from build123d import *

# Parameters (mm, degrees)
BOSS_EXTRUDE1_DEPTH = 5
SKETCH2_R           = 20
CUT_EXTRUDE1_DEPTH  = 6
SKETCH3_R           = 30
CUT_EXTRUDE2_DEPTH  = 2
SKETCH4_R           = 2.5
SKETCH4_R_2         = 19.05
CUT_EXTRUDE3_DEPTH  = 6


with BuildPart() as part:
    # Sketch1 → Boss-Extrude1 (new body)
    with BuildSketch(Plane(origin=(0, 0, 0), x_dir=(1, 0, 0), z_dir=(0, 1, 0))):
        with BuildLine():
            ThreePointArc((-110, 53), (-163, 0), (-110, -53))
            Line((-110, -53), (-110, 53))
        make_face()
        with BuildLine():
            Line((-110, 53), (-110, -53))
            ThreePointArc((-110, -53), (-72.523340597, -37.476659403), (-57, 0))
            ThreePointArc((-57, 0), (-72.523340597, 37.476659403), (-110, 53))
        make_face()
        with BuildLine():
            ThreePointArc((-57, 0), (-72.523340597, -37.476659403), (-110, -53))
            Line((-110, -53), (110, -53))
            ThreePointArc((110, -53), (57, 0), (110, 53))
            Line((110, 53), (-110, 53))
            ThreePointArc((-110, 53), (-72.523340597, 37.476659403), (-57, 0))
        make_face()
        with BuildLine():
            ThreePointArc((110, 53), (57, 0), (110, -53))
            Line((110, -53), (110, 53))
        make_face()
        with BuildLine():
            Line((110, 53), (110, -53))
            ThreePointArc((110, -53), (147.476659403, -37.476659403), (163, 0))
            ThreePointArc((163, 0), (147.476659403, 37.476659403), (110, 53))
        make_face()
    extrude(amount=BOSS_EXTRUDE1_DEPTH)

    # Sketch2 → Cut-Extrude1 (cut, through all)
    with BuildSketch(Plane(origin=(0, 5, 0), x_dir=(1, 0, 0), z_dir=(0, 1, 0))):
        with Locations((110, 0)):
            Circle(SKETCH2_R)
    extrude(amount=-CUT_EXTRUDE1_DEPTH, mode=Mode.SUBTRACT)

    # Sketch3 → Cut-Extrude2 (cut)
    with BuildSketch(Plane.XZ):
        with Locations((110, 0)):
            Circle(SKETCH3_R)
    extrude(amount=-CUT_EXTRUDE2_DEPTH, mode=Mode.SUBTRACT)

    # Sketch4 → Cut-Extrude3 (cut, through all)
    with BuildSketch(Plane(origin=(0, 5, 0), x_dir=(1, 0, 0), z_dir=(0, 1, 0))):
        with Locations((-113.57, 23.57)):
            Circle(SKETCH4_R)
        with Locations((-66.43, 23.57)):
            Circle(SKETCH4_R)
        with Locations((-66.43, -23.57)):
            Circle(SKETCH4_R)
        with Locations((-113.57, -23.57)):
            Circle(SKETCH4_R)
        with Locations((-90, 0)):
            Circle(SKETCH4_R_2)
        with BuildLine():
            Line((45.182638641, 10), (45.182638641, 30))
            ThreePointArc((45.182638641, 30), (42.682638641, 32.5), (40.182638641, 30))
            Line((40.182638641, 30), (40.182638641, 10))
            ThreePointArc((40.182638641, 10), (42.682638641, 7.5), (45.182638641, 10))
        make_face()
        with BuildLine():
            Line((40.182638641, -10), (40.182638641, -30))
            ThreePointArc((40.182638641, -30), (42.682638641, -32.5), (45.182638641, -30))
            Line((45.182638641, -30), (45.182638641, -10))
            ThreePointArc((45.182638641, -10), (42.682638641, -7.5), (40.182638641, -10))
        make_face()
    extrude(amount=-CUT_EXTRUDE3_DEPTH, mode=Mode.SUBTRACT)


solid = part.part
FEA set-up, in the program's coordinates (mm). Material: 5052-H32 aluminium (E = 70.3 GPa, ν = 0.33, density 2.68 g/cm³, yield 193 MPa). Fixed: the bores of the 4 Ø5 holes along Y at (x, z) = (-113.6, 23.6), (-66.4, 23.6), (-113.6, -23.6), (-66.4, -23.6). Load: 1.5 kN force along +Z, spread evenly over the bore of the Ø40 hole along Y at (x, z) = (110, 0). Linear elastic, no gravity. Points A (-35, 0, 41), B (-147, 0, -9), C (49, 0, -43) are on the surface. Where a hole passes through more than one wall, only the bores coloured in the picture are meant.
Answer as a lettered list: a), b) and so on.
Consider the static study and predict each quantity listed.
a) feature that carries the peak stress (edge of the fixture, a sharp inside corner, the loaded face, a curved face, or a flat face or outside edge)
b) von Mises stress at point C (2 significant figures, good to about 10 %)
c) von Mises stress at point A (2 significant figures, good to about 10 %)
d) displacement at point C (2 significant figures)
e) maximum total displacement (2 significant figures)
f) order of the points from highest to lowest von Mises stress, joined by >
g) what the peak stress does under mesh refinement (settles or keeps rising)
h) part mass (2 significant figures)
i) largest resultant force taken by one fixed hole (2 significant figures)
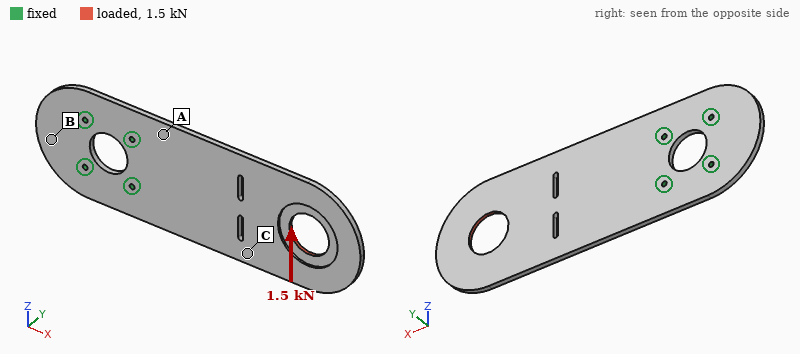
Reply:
a) edge of the fixture
b) 7.7 MPa
c) 18 MPa
d) 0.10 mm
e) 0.20 mm
f) A > C > B
g) keeps rising
h) 390 g
i) 3.3 kN
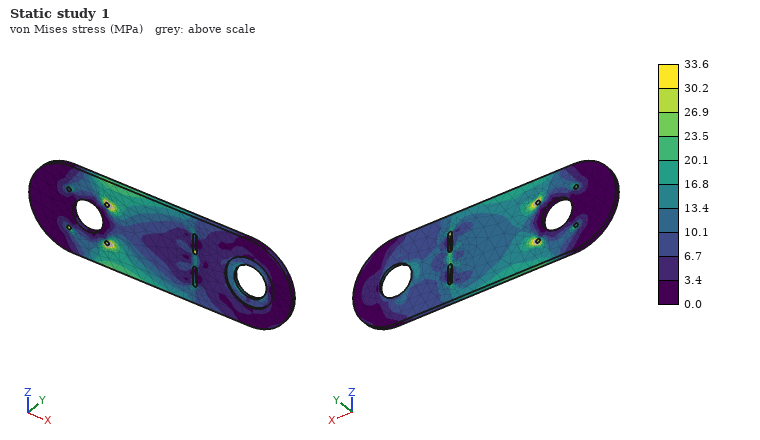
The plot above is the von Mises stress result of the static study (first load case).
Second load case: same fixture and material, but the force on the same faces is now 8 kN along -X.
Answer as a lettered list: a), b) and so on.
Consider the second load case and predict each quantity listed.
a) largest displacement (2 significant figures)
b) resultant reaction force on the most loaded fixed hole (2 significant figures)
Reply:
a) 2.8 mm
b) 3.3 kN
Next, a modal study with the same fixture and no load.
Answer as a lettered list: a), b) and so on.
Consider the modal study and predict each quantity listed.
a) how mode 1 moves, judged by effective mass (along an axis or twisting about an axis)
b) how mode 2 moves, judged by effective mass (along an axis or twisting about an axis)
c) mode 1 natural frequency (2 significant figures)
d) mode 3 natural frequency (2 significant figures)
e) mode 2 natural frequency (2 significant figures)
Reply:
a) along Y
b) twisting about X
c) 93 Hz
d) 480 Hz
e) 380 Hz
